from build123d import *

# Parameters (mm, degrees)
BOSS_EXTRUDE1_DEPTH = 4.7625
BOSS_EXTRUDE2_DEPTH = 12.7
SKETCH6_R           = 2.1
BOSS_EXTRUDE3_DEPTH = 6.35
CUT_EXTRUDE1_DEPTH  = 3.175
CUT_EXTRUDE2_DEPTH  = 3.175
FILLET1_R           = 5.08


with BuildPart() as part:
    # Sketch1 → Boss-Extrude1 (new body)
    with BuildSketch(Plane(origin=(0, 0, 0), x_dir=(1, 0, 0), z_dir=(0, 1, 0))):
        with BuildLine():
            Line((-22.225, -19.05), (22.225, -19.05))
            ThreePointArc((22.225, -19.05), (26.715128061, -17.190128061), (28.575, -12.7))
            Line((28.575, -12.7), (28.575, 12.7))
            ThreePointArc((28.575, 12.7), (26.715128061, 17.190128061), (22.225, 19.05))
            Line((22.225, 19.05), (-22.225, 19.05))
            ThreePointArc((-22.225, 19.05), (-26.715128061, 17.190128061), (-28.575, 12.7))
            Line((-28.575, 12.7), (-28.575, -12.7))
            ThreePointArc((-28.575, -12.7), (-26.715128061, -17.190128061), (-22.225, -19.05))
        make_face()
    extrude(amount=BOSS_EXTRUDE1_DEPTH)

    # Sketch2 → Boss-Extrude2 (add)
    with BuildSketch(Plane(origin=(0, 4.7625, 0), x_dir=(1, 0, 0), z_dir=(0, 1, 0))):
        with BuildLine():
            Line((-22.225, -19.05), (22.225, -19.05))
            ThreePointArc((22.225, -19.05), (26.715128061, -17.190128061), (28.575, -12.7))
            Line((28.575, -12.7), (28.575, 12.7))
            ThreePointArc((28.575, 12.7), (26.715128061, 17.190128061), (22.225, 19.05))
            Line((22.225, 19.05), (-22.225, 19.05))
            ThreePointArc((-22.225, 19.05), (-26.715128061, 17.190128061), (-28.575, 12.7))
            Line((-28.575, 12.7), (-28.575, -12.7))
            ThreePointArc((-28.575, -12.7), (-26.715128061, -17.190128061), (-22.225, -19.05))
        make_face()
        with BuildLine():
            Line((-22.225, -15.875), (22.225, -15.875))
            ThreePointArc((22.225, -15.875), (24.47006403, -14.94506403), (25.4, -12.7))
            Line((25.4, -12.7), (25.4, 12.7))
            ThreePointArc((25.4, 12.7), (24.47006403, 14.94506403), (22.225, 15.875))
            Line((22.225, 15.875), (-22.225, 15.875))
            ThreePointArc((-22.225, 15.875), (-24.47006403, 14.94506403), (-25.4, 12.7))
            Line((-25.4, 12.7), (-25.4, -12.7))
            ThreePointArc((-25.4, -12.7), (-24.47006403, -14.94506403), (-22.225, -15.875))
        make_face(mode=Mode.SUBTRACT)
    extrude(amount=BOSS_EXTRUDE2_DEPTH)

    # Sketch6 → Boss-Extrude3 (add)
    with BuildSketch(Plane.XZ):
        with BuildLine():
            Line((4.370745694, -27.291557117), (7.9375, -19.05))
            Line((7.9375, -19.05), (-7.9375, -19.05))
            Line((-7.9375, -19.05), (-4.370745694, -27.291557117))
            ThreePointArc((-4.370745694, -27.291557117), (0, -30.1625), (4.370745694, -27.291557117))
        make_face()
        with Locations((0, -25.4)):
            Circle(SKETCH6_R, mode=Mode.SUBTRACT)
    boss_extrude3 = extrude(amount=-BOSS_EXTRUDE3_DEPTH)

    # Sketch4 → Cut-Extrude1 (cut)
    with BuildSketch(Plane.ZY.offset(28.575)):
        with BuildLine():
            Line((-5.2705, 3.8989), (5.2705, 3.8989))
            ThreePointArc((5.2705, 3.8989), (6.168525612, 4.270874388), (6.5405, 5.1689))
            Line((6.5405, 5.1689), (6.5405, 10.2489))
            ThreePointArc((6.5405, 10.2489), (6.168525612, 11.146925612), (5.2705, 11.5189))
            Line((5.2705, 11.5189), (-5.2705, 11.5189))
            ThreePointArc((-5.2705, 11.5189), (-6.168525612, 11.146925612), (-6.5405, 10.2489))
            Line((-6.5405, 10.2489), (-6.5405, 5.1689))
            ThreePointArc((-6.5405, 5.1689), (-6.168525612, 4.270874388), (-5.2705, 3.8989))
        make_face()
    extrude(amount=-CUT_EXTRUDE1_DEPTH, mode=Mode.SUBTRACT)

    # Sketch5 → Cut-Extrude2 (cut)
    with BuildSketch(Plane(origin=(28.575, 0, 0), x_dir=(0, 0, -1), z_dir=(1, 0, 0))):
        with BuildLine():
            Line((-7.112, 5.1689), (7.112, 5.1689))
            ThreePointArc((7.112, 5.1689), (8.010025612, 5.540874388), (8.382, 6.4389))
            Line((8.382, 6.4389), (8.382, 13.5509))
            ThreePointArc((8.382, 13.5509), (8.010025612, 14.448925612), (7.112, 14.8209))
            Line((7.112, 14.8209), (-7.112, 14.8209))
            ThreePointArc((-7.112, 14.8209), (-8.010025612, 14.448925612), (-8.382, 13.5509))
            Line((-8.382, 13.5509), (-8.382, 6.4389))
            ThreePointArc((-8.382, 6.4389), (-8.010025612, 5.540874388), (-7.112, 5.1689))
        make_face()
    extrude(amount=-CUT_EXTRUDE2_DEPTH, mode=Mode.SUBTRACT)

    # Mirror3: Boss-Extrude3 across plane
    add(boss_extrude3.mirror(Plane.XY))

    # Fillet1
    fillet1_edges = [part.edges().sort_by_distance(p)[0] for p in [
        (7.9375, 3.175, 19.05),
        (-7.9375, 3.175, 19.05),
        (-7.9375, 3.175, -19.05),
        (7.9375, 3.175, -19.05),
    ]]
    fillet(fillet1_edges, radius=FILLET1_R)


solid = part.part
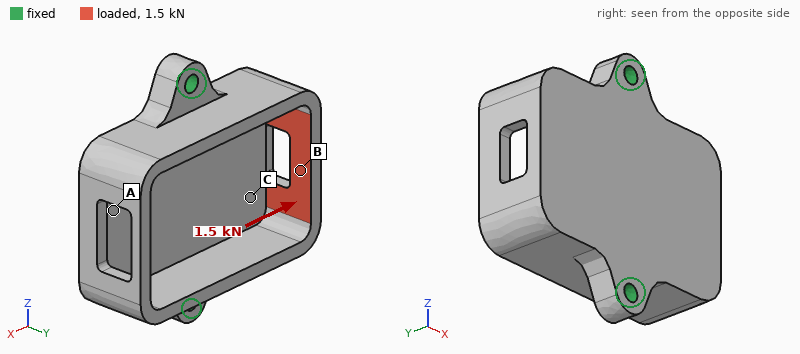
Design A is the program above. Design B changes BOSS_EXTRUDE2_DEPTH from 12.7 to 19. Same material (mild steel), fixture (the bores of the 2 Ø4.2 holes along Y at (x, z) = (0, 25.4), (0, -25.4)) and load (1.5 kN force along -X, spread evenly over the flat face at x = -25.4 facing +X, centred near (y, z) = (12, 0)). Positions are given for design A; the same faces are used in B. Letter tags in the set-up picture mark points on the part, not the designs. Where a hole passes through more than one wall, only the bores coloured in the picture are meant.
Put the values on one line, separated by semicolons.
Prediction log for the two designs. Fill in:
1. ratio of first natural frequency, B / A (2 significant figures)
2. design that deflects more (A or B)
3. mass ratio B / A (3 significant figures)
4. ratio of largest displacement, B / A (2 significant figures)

0.84; B; 1.19; 1.1
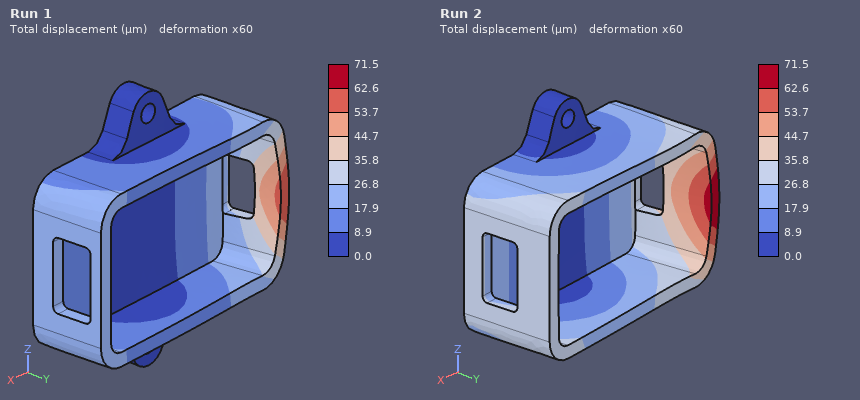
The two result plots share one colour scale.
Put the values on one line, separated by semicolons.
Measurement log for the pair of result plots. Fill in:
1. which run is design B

Run 2
